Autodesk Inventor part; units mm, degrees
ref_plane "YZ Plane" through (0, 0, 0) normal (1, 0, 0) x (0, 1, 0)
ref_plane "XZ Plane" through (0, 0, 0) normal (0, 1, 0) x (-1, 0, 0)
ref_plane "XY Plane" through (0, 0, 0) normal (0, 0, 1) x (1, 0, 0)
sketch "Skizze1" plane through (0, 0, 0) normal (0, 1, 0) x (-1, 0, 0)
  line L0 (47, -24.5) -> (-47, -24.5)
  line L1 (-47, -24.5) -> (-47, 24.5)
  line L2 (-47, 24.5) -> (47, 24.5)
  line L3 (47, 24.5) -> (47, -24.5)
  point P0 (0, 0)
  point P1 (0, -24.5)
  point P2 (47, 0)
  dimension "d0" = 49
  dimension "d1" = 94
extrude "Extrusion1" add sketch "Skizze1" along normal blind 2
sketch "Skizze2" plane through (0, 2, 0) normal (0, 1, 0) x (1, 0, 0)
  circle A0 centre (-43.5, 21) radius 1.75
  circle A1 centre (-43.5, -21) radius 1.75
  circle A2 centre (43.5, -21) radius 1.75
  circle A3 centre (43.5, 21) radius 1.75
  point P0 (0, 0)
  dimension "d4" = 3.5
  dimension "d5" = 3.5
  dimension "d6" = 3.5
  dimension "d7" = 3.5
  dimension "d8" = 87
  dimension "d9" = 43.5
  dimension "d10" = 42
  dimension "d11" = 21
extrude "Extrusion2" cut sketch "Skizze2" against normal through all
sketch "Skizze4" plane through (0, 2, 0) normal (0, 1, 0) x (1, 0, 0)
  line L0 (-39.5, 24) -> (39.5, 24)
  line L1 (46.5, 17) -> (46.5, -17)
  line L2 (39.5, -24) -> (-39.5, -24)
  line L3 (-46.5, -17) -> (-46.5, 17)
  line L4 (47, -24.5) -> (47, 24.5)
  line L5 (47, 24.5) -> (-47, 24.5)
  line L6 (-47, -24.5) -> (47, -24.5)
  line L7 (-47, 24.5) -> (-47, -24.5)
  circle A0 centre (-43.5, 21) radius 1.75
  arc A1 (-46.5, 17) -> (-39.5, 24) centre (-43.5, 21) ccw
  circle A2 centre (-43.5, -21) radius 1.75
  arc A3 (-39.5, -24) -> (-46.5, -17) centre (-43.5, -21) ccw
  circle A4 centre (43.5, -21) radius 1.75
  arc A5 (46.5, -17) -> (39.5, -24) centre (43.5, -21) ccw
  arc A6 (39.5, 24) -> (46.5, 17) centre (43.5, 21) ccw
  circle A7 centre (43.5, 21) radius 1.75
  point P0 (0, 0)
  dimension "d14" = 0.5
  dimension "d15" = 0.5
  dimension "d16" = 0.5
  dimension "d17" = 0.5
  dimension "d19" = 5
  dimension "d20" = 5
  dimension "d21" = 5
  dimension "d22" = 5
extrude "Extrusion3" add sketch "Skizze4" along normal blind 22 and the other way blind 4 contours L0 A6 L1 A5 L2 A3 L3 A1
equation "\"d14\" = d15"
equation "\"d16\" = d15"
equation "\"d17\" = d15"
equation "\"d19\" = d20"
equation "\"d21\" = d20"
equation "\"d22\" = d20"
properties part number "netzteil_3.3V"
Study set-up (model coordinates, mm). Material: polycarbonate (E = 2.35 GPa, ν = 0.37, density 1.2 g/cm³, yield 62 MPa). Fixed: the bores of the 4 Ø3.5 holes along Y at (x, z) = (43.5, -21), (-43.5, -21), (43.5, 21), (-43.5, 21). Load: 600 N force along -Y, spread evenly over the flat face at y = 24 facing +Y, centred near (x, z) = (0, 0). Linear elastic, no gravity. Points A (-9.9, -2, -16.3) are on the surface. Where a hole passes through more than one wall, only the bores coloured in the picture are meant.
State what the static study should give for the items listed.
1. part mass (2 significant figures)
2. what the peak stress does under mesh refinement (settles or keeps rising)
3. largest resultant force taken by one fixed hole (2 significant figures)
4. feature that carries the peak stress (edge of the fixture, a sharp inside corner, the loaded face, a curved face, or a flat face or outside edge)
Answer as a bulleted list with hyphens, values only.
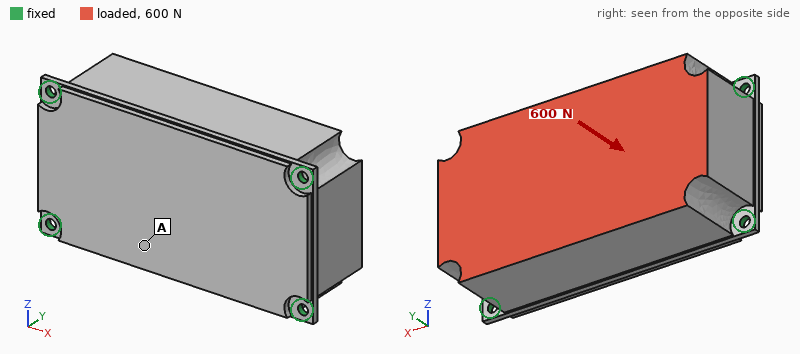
- 130 g
- keeps rising
- 160 N
- edge of the fixture
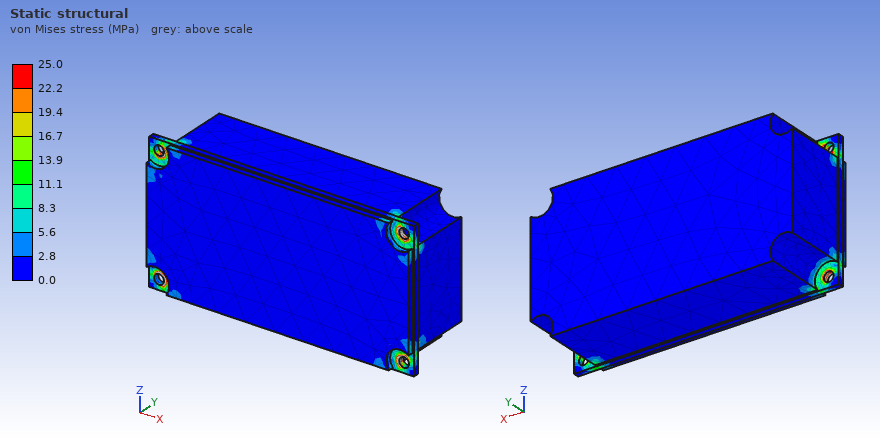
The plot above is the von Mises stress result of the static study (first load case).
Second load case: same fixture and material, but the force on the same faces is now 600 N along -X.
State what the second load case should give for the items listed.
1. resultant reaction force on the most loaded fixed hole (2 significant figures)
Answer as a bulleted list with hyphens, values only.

- 180 N
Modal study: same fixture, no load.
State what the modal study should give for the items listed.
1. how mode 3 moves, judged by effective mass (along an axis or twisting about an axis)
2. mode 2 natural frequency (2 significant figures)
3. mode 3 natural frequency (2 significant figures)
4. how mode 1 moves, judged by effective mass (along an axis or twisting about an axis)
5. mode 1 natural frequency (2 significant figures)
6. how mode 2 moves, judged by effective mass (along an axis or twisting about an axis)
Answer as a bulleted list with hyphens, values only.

- along X
- 1200 Hz
- 1700 Hz
- along Y
- 1100 Hz
- along Z
